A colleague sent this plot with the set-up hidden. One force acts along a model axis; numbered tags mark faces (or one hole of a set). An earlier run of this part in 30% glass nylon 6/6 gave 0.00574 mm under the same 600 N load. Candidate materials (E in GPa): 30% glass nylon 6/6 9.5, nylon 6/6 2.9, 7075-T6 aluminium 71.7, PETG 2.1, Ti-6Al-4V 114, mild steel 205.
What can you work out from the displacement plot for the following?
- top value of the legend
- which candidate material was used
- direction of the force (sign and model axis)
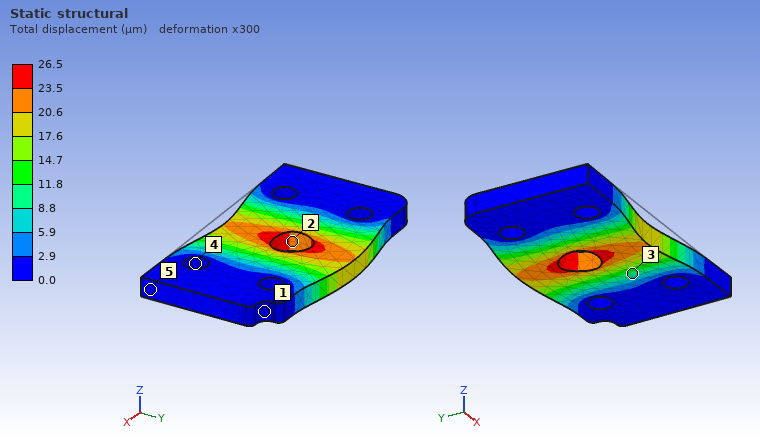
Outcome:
26.5 µm
PETG
+Y
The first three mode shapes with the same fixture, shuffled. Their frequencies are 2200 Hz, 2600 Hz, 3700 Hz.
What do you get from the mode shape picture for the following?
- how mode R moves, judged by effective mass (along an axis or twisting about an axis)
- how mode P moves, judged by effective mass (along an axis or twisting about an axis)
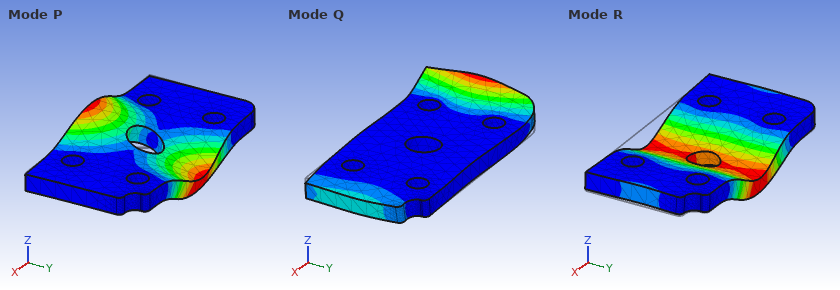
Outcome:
along Z
twisting about X
